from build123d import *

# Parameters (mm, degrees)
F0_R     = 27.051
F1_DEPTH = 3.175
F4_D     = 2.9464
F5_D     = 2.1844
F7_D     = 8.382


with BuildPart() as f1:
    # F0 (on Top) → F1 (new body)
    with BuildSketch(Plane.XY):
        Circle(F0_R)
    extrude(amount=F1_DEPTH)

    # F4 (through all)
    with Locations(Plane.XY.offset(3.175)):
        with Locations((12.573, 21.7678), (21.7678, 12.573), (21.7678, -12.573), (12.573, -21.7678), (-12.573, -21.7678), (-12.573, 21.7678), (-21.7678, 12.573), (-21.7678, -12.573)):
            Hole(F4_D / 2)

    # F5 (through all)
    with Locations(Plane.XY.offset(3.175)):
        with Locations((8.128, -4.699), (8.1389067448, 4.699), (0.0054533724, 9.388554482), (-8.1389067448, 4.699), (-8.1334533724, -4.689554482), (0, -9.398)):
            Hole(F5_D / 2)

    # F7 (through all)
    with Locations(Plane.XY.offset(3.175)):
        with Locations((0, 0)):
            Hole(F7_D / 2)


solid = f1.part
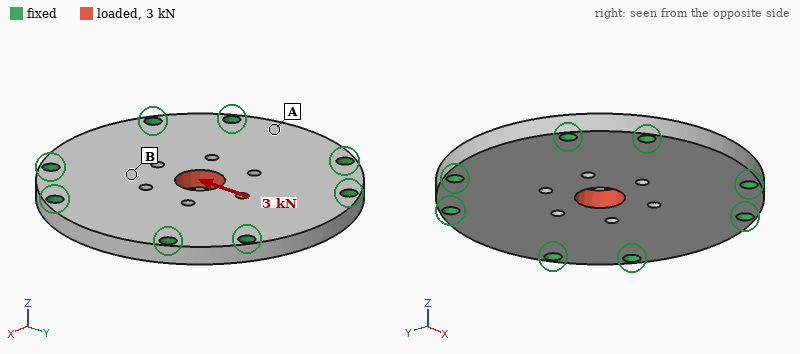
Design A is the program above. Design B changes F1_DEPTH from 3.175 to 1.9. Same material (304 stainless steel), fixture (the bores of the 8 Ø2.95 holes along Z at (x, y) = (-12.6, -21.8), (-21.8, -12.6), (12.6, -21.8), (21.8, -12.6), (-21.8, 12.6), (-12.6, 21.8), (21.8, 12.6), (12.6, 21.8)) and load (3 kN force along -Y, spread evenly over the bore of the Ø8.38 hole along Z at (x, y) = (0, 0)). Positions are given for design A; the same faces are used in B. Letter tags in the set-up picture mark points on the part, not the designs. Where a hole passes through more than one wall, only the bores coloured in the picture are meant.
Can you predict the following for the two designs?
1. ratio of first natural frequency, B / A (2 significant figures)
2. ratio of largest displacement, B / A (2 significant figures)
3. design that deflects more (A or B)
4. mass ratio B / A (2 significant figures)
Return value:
0.64
1.7
B
0.60
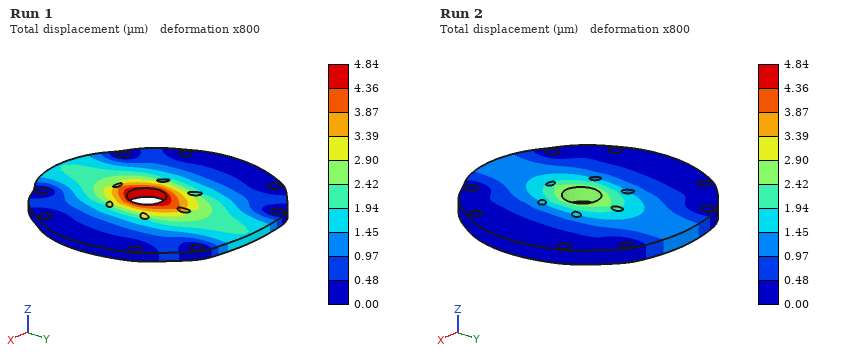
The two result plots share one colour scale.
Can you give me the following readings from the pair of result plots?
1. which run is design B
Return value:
Run 1
